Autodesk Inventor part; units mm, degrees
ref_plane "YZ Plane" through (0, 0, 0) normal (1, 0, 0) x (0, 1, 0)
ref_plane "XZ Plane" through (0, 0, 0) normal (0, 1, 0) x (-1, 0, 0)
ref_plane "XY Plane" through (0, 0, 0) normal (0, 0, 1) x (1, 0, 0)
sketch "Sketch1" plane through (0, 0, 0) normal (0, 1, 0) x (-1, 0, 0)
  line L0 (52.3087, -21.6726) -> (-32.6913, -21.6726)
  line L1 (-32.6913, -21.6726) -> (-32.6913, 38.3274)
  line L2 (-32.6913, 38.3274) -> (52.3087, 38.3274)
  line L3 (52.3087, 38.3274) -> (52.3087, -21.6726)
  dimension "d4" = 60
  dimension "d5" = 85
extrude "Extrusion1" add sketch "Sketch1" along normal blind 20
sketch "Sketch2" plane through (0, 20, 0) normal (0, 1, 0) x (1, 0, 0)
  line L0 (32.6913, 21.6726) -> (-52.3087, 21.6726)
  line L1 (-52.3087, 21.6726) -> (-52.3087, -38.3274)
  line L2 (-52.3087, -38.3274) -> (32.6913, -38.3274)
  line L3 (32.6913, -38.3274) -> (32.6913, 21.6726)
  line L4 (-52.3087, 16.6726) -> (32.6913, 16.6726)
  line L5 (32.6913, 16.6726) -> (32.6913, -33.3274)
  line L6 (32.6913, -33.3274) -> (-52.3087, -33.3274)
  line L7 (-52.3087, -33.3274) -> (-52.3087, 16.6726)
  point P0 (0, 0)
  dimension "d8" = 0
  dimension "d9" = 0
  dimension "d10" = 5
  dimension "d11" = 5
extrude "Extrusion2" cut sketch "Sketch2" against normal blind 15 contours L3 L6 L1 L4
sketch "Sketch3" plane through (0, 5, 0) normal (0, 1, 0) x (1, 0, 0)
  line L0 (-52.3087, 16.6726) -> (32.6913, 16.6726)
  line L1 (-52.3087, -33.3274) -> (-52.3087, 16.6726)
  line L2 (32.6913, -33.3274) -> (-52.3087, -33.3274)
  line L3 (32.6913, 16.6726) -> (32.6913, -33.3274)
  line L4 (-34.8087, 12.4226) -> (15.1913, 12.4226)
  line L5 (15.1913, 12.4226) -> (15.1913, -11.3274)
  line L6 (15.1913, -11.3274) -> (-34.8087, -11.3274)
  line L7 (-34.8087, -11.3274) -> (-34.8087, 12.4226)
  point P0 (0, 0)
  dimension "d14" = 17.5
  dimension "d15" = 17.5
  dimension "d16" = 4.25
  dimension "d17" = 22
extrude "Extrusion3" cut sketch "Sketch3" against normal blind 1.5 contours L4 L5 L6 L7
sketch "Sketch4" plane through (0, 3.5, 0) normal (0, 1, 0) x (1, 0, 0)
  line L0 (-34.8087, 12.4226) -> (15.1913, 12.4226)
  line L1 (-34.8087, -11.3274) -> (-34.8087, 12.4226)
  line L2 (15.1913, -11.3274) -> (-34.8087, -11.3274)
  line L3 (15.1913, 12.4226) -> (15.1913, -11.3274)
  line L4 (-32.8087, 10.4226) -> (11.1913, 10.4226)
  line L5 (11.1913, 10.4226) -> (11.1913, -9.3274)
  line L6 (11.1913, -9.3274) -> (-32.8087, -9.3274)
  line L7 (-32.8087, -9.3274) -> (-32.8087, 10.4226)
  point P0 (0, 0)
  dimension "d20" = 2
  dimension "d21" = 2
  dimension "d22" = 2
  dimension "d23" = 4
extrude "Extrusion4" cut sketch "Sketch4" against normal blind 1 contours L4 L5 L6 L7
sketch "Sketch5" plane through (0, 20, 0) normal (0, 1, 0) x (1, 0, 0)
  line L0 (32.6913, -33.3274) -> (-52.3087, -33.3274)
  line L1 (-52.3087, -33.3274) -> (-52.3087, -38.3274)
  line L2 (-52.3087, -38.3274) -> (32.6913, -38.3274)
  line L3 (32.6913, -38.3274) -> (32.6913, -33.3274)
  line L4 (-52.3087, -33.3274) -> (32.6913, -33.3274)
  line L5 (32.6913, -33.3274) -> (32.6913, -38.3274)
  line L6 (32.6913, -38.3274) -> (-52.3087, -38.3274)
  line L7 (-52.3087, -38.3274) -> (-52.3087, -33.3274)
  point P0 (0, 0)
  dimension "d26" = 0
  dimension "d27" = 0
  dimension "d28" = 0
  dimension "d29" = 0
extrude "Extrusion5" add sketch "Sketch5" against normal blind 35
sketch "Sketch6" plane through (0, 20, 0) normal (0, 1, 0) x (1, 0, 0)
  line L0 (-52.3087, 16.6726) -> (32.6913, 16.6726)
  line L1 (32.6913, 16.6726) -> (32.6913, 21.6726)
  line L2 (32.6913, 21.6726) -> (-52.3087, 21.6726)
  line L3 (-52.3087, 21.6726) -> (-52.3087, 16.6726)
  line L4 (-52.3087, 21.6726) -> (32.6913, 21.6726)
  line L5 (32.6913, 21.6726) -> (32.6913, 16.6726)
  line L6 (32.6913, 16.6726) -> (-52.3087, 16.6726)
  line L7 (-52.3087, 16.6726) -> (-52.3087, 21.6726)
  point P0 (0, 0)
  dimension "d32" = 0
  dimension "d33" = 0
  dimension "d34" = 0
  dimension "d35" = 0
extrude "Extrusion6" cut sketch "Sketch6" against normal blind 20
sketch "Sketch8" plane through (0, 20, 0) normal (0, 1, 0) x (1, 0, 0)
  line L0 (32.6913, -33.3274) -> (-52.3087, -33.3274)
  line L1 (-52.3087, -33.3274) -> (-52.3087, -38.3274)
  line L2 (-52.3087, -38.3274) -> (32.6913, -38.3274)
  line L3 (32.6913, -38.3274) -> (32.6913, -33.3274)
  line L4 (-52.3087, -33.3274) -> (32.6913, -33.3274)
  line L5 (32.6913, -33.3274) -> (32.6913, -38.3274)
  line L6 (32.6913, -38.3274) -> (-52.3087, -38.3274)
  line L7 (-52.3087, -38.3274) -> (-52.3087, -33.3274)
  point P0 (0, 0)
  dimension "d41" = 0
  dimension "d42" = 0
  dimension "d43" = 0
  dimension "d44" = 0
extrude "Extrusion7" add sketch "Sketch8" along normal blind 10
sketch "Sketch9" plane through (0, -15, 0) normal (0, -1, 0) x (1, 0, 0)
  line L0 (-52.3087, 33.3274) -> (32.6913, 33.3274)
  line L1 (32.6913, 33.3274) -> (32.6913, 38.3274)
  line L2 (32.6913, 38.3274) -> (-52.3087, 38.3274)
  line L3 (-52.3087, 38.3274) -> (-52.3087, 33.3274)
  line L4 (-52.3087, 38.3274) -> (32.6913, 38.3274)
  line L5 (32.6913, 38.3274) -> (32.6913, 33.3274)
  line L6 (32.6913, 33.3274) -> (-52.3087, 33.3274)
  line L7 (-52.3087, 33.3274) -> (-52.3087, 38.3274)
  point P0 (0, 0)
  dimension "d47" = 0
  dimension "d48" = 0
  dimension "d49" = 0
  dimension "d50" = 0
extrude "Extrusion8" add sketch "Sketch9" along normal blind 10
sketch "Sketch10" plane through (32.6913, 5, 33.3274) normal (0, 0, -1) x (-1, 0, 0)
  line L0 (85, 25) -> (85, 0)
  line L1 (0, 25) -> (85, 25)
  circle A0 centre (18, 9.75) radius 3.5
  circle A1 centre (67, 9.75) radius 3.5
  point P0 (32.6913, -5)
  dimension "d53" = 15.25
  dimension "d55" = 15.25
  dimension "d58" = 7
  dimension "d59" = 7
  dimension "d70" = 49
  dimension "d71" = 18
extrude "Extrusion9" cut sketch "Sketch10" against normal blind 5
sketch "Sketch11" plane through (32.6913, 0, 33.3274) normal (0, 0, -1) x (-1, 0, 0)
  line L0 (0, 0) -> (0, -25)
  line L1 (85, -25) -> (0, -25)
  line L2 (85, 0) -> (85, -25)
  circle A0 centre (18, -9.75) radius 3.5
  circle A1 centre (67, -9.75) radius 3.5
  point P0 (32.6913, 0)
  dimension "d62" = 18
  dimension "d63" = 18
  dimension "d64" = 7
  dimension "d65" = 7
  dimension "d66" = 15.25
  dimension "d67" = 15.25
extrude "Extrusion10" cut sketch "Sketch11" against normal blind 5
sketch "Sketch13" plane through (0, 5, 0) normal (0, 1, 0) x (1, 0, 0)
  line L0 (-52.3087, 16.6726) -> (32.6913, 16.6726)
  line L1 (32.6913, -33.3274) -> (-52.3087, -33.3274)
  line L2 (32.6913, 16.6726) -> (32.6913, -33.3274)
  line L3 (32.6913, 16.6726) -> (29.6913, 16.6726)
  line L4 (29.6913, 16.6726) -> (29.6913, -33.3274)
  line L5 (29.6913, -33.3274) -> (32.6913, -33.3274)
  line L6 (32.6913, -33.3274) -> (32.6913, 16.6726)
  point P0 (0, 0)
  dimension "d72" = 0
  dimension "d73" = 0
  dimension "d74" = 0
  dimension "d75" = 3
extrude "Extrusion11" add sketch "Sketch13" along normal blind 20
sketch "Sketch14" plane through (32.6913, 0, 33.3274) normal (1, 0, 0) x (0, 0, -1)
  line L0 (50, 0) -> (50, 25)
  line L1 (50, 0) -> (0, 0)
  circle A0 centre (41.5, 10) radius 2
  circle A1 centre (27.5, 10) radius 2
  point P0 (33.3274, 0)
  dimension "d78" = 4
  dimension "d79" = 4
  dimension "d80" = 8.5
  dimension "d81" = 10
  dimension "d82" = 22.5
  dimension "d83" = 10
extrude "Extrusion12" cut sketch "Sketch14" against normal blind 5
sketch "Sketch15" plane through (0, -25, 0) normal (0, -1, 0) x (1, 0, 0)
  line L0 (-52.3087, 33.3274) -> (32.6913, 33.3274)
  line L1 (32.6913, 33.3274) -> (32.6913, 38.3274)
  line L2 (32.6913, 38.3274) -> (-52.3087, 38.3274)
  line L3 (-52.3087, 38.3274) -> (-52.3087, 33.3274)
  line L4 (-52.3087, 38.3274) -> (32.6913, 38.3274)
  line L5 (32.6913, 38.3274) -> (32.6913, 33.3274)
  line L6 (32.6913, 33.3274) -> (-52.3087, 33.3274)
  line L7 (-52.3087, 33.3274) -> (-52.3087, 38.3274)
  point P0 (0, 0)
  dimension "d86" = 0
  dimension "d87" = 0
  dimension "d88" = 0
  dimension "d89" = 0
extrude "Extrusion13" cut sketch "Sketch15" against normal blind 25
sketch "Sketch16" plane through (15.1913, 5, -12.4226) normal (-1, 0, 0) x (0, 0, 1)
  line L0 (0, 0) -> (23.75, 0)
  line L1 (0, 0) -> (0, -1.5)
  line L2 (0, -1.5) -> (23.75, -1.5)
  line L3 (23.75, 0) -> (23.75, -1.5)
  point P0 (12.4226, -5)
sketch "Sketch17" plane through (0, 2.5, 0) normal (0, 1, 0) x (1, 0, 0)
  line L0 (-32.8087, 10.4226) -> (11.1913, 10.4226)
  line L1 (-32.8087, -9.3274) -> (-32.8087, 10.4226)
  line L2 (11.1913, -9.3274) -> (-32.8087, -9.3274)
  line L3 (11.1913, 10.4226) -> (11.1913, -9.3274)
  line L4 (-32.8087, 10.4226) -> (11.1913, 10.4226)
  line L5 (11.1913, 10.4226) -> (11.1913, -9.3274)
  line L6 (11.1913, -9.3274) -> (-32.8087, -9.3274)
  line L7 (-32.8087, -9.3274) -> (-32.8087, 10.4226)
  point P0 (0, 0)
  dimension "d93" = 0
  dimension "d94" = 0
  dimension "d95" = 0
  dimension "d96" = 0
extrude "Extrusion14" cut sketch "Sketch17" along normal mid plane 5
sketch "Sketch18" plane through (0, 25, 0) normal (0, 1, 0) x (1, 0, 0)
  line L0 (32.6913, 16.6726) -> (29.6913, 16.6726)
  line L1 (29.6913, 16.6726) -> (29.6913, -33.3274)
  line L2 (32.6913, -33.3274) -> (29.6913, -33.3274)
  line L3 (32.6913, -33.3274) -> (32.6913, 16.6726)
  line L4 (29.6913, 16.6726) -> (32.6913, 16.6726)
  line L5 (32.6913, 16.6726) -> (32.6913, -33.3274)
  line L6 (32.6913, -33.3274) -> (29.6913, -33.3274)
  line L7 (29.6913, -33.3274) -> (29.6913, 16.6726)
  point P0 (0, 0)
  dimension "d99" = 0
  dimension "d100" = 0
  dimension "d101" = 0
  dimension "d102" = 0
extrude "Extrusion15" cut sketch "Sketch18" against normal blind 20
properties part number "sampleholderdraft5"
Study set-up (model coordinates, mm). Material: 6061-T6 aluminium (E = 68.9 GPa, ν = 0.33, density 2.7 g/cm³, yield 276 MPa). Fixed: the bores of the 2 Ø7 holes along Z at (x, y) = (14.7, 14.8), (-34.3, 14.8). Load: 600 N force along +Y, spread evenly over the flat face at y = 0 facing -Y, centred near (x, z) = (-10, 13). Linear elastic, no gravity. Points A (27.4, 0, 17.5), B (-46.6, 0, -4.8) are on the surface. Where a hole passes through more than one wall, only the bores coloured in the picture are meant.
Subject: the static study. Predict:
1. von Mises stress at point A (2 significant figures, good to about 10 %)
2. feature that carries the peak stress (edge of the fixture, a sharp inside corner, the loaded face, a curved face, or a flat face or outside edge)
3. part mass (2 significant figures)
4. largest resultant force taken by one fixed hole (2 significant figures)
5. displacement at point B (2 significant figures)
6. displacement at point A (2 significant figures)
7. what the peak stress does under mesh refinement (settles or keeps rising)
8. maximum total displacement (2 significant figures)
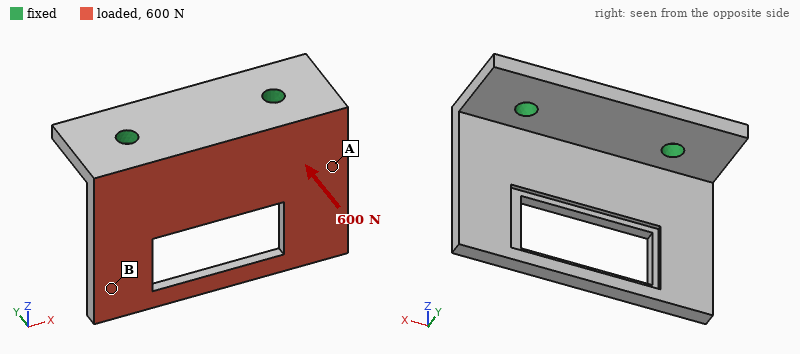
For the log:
22 MPa
edge of the fixture
78 g
300 N
0.22 mm
0.080 mm
keeps rising
0.31 mm
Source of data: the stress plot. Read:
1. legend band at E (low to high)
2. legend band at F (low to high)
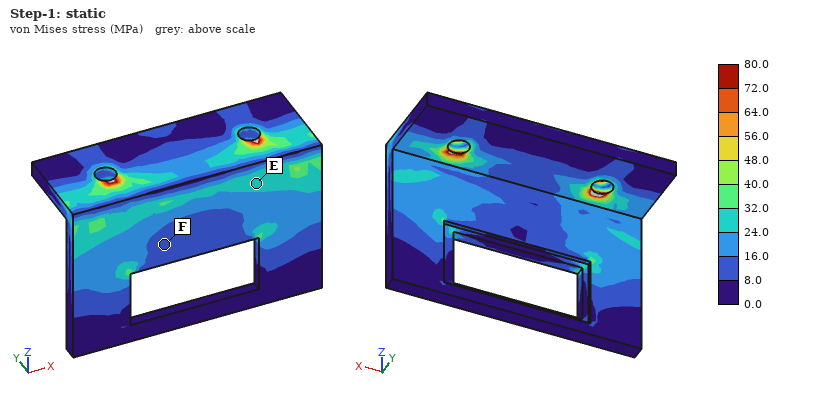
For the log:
24.0 to 32.0 MPa
8.0 to 16.0 MPa
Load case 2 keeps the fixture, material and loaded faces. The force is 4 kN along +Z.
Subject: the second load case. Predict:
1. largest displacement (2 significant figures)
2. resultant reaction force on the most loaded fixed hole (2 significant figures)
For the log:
0.53 mm
2.0 kN
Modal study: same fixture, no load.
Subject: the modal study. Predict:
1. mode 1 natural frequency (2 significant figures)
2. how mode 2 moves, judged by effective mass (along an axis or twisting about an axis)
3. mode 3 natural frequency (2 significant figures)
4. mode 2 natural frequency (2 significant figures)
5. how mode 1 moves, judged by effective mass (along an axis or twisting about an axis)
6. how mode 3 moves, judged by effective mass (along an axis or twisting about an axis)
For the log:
1200 Hz
twisting about Z
4500 Hz
1900 Hz
along Y
along X
